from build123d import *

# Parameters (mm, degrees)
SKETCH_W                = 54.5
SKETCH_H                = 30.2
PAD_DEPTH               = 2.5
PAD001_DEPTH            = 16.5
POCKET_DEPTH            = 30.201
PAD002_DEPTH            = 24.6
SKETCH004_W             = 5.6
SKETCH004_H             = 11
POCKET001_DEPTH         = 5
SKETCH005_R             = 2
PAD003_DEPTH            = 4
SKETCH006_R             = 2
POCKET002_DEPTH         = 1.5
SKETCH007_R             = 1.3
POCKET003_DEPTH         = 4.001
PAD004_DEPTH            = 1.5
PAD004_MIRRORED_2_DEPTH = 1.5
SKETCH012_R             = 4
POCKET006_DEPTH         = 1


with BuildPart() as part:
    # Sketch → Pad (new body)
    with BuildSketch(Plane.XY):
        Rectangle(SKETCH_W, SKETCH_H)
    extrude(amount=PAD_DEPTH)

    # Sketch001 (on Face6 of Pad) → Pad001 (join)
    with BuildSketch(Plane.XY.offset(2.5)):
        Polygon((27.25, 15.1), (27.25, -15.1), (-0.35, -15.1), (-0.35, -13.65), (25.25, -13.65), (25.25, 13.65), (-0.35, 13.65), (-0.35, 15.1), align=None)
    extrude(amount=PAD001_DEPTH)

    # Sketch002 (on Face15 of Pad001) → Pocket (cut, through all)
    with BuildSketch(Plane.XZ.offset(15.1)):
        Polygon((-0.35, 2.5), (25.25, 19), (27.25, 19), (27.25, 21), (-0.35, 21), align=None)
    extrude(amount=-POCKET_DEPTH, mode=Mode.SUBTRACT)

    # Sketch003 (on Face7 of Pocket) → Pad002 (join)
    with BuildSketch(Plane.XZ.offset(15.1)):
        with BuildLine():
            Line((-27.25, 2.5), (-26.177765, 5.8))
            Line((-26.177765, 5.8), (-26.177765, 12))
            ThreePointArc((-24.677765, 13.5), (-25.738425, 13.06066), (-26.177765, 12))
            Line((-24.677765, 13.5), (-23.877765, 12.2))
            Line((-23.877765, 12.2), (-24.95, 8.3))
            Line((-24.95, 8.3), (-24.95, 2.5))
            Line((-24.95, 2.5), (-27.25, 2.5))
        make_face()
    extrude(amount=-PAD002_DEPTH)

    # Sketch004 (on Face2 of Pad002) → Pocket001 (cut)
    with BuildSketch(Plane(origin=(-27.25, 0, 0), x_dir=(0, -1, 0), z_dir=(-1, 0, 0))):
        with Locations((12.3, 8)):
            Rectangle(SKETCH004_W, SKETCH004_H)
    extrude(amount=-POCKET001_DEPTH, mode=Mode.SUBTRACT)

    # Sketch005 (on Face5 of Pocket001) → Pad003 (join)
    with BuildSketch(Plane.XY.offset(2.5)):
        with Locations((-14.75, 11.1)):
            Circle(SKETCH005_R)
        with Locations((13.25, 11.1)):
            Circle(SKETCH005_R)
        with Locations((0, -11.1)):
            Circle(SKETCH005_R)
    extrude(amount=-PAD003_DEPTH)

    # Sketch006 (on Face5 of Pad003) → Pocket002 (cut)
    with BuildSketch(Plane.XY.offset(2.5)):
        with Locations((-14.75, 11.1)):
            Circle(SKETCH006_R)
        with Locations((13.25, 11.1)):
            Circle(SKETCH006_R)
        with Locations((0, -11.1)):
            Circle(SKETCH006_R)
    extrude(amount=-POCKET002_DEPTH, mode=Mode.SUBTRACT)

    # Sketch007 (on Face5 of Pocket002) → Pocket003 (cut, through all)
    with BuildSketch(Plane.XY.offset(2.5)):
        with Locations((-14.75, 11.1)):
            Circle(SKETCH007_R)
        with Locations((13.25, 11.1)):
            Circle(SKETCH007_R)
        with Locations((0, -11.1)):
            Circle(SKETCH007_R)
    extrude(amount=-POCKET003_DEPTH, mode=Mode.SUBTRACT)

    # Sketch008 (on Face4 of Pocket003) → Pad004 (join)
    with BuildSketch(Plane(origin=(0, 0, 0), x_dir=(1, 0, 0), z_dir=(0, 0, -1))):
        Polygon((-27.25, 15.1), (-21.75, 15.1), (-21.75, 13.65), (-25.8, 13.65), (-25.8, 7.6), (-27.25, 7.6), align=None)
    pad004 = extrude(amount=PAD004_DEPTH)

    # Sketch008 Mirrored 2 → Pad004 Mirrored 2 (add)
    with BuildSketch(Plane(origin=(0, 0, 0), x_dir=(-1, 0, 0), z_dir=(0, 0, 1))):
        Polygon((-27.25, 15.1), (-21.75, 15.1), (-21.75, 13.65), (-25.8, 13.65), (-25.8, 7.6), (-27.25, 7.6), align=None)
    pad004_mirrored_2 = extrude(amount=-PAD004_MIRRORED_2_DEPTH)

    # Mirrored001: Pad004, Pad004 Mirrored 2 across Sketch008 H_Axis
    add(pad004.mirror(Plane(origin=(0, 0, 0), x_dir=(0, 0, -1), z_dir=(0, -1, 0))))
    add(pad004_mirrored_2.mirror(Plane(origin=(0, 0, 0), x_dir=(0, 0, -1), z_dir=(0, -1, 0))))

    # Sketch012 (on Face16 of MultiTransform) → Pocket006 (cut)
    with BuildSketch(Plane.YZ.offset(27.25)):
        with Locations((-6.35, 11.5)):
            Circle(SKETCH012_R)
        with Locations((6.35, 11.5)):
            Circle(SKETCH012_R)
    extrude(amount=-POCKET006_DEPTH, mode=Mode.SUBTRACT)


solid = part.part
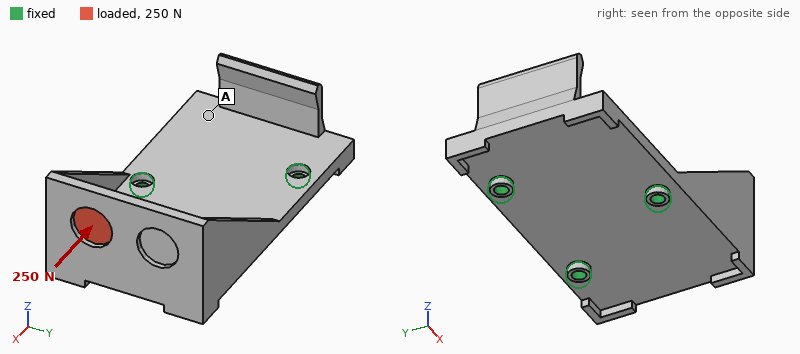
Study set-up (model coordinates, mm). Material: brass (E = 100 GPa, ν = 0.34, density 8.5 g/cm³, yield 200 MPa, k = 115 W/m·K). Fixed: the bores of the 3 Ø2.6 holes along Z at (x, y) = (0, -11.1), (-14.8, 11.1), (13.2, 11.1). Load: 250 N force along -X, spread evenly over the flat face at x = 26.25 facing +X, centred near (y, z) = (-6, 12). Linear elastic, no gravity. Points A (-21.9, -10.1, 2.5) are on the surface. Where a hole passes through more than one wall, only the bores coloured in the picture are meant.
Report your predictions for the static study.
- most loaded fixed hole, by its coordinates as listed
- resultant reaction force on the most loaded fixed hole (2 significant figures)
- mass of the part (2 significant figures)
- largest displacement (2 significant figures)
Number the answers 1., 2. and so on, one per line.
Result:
1. (-14.8, 11.1)
2. 210 N
3. 51 g
4. 0.14 mm
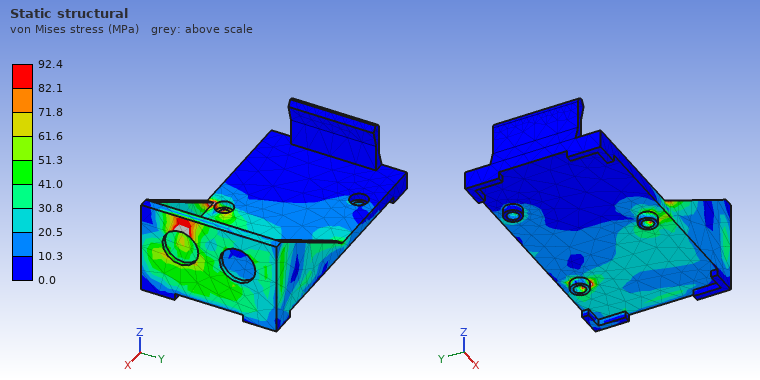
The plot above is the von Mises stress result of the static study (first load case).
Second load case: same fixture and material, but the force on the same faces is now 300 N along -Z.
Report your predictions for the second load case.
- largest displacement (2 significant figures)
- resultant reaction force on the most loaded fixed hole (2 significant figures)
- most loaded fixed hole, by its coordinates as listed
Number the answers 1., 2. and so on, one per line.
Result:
1. 0.34 mm
2. 460 N
3. (-14.8, 11.1)
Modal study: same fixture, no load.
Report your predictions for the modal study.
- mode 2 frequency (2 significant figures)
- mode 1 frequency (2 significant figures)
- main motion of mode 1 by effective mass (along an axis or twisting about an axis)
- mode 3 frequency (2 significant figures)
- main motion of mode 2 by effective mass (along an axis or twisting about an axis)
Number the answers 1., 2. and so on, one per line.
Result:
1. 2200 Hz
2. 1700 Hz
3. along Z
4. 4000 Hz
5. along Z
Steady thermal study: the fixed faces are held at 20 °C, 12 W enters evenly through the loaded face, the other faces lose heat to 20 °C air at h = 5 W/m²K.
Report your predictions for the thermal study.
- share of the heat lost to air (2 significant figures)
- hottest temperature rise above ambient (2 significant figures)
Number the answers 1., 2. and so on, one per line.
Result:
1. 3.3 %
2. 50 K
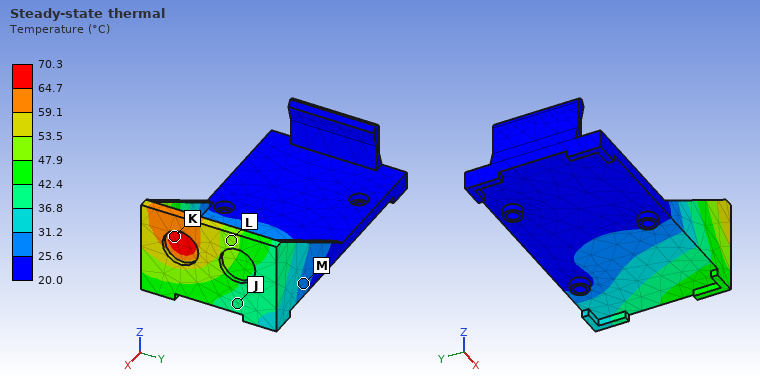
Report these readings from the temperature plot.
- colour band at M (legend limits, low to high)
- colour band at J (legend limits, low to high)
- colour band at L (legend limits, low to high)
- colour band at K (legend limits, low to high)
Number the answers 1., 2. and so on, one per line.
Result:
1. 25.6 to 31.2 °C
2. 36.8 to 42.4 °C
3. 47.9 to 53.5 °C
4. 64.7 to 70.3 °C
